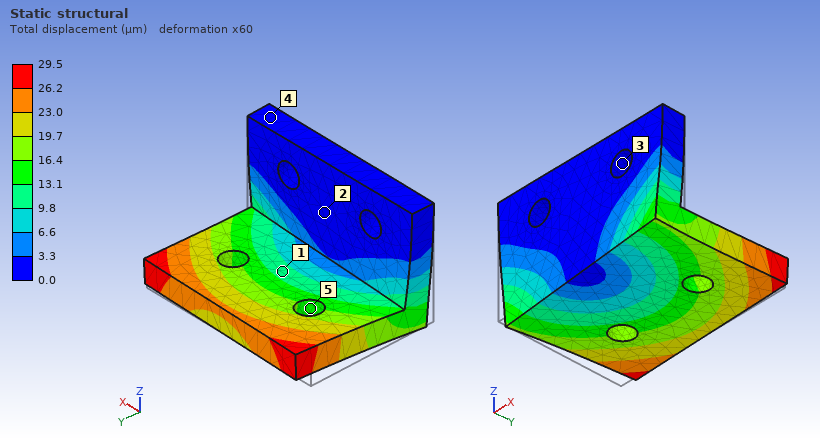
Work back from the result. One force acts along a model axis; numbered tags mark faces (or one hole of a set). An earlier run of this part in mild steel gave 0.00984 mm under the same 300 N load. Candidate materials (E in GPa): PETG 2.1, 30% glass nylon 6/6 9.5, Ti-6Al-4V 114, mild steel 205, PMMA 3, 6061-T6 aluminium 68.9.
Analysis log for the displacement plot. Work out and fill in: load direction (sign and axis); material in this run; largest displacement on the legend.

+X
6061-T6 aluminium
29.5 µm
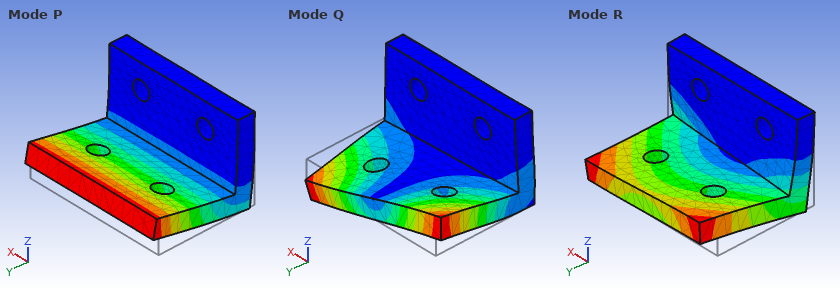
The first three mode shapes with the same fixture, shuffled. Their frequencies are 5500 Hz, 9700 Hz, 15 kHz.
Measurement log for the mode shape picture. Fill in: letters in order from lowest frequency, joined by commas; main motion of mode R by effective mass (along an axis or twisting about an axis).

P, R, Q
along X
